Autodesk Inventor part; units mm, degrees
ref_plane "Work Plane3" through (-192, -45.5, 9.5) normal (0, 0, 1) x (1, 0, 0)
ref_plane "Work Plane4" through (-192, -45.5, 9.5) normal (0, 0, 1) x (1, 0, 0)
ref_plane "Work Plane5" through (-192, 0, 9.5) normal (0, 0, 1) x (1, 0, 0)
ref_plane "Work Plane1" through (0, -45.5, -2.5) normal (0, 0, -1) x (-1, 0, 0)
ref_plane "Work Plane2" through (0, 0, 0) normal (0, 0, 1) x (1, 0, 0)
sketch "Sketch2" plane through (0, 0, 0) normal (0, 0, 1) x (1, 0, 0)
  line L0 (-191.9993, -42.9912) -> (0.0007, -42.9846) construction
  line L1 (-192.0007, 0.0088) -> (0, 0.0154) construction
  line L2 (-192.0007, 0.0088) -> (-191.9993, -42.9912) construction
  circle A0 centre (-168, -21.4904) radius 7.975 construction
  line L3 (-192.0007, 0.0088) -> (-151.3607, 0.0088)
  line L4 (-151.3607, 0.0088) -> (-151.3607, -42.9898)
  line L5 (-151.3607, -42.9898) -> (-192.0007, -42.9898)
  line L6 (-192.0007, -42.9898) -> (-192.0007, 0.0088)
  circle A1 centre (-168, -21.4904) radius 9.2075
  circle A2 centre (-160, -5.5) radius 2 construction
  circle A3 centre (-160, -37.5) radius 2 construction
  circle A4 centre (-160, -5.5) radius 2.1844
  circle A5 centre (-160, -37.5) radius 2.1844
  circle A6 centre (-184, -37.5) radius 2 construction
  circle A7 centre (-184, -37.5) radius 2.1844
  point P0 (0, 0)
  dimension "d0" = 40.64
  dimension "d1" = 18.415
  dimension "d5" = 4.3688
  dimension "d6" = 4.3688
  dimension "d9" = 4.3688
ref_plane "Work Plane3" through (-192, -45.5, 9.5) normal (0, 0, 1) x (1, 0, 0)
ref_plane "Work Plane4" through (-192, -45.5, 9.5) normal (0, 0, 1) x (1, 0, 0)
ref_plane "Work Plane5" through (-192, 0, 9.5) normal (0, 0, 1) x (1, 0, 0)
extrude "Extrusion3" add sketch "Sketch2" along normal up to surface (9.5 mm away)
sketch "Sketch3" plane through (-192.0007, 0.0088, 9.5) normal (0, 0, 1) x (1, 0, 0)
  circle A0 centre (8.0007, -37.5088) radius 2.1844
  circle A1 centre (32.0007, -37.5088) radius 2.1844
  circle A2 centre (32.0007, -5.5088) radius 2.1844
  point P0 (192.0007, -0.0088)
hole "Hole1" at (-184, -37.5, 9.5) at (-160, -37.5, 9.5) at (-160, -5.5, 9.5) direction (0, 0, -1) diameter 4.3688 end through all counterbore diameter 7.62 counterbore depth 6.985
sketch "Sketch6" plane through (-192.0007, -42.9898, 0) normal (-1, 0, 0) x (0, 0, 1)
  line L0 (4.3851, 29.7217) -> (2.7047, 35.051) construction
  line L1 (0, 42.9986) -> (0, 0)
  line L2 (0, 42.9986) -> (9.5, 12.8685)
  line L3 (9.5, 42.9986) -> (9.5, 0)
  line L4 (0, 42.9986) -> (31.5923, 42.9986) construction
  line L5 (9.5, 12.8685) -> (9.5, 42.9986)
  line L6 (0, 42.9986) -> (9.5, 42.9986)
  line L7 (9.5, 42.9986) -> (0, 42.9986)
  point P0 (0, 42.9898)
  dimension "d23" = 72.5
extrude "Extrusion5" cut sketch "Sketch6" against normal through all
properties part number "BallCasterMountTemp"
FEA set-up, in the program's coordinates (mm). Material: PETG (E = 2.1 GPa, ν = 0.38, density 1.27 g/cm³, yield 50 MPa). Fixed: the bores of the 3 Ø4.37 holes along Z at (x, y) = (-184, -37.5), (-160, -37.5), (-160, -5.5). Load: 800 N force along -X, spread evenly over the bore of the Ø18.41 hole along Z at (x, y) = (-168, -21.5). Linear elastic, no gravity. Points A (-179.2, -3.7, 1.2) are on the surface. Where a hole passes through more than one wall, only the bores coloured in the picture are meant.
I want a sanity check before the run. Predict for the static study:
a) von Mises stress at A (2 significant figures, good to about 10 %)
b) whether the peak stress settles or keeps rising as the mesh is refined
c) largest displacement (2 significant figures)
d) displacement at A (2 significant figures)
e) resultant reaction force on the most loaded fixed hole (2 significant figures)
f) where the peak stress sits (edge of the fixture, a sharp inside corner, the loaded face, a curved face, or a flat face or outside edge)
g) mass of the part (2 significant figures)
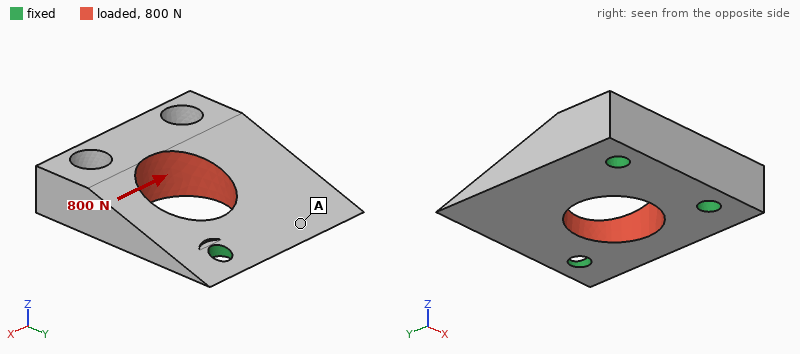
3.2 MPa
keeps rising
91 µm
62 µm
300 N
edge of the fixture
10 g
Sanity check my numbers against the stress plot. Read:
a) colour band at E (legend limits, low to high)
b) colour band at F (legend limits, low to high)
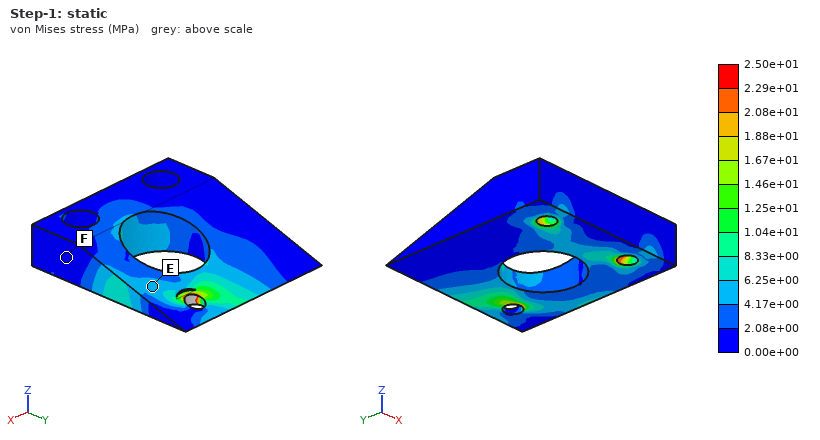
4.17e+00 to 6.25e+00 MPa
0.00e+00 to 2.08e+00 MPa
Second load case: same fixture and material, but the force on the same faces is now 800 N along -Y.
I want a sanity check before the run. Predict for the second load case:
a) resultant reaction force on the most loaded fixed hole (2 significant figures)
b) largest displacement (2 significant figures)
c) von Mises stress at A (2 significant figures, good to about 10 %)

310 N
0.24 mm
2.9 MPa
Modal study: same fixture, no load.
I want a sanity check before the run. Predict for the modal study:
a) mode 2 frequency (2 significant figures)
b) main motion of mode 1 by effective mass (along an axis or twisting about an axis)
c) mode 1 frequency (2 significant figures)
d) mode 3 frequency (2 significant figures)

4300 Hz
along Z
1700 Hz
4700 Hz
